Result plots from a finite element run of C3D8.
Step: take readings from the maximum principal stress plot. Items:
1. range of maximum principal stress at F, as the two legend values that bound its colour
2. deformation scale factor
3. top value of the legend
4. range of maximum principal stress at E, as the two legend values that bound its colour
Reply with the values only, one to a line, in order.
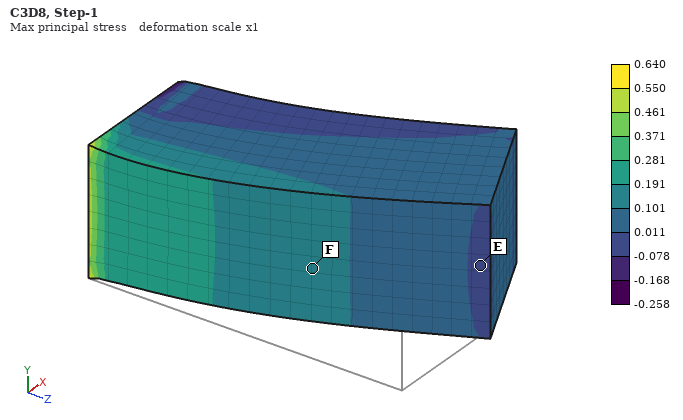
0.101 to 0.191
1
0.640
-0.078 to 0.011
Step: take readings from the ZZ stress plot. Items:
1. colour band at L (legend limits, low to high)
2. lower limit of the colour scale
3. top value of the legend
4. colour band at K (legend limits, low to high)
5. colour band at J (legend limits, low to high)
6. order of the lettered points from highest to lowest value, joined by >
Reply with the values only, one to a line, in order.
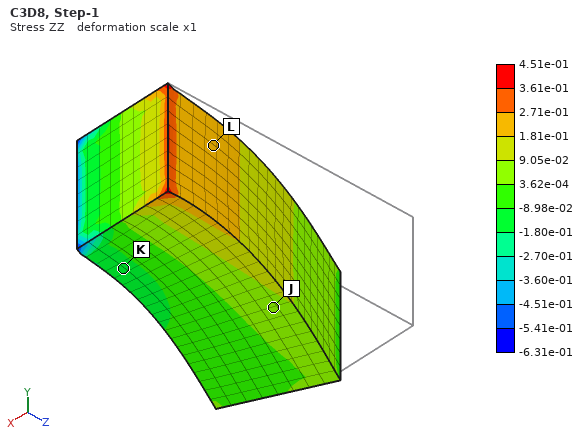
1.81e-01 to 2.71e-01
-6.31e-01
4.51e-01
-1.80e-01 to -8.98e-02
3.62e-04 to 9.05e-02
L > J > K
